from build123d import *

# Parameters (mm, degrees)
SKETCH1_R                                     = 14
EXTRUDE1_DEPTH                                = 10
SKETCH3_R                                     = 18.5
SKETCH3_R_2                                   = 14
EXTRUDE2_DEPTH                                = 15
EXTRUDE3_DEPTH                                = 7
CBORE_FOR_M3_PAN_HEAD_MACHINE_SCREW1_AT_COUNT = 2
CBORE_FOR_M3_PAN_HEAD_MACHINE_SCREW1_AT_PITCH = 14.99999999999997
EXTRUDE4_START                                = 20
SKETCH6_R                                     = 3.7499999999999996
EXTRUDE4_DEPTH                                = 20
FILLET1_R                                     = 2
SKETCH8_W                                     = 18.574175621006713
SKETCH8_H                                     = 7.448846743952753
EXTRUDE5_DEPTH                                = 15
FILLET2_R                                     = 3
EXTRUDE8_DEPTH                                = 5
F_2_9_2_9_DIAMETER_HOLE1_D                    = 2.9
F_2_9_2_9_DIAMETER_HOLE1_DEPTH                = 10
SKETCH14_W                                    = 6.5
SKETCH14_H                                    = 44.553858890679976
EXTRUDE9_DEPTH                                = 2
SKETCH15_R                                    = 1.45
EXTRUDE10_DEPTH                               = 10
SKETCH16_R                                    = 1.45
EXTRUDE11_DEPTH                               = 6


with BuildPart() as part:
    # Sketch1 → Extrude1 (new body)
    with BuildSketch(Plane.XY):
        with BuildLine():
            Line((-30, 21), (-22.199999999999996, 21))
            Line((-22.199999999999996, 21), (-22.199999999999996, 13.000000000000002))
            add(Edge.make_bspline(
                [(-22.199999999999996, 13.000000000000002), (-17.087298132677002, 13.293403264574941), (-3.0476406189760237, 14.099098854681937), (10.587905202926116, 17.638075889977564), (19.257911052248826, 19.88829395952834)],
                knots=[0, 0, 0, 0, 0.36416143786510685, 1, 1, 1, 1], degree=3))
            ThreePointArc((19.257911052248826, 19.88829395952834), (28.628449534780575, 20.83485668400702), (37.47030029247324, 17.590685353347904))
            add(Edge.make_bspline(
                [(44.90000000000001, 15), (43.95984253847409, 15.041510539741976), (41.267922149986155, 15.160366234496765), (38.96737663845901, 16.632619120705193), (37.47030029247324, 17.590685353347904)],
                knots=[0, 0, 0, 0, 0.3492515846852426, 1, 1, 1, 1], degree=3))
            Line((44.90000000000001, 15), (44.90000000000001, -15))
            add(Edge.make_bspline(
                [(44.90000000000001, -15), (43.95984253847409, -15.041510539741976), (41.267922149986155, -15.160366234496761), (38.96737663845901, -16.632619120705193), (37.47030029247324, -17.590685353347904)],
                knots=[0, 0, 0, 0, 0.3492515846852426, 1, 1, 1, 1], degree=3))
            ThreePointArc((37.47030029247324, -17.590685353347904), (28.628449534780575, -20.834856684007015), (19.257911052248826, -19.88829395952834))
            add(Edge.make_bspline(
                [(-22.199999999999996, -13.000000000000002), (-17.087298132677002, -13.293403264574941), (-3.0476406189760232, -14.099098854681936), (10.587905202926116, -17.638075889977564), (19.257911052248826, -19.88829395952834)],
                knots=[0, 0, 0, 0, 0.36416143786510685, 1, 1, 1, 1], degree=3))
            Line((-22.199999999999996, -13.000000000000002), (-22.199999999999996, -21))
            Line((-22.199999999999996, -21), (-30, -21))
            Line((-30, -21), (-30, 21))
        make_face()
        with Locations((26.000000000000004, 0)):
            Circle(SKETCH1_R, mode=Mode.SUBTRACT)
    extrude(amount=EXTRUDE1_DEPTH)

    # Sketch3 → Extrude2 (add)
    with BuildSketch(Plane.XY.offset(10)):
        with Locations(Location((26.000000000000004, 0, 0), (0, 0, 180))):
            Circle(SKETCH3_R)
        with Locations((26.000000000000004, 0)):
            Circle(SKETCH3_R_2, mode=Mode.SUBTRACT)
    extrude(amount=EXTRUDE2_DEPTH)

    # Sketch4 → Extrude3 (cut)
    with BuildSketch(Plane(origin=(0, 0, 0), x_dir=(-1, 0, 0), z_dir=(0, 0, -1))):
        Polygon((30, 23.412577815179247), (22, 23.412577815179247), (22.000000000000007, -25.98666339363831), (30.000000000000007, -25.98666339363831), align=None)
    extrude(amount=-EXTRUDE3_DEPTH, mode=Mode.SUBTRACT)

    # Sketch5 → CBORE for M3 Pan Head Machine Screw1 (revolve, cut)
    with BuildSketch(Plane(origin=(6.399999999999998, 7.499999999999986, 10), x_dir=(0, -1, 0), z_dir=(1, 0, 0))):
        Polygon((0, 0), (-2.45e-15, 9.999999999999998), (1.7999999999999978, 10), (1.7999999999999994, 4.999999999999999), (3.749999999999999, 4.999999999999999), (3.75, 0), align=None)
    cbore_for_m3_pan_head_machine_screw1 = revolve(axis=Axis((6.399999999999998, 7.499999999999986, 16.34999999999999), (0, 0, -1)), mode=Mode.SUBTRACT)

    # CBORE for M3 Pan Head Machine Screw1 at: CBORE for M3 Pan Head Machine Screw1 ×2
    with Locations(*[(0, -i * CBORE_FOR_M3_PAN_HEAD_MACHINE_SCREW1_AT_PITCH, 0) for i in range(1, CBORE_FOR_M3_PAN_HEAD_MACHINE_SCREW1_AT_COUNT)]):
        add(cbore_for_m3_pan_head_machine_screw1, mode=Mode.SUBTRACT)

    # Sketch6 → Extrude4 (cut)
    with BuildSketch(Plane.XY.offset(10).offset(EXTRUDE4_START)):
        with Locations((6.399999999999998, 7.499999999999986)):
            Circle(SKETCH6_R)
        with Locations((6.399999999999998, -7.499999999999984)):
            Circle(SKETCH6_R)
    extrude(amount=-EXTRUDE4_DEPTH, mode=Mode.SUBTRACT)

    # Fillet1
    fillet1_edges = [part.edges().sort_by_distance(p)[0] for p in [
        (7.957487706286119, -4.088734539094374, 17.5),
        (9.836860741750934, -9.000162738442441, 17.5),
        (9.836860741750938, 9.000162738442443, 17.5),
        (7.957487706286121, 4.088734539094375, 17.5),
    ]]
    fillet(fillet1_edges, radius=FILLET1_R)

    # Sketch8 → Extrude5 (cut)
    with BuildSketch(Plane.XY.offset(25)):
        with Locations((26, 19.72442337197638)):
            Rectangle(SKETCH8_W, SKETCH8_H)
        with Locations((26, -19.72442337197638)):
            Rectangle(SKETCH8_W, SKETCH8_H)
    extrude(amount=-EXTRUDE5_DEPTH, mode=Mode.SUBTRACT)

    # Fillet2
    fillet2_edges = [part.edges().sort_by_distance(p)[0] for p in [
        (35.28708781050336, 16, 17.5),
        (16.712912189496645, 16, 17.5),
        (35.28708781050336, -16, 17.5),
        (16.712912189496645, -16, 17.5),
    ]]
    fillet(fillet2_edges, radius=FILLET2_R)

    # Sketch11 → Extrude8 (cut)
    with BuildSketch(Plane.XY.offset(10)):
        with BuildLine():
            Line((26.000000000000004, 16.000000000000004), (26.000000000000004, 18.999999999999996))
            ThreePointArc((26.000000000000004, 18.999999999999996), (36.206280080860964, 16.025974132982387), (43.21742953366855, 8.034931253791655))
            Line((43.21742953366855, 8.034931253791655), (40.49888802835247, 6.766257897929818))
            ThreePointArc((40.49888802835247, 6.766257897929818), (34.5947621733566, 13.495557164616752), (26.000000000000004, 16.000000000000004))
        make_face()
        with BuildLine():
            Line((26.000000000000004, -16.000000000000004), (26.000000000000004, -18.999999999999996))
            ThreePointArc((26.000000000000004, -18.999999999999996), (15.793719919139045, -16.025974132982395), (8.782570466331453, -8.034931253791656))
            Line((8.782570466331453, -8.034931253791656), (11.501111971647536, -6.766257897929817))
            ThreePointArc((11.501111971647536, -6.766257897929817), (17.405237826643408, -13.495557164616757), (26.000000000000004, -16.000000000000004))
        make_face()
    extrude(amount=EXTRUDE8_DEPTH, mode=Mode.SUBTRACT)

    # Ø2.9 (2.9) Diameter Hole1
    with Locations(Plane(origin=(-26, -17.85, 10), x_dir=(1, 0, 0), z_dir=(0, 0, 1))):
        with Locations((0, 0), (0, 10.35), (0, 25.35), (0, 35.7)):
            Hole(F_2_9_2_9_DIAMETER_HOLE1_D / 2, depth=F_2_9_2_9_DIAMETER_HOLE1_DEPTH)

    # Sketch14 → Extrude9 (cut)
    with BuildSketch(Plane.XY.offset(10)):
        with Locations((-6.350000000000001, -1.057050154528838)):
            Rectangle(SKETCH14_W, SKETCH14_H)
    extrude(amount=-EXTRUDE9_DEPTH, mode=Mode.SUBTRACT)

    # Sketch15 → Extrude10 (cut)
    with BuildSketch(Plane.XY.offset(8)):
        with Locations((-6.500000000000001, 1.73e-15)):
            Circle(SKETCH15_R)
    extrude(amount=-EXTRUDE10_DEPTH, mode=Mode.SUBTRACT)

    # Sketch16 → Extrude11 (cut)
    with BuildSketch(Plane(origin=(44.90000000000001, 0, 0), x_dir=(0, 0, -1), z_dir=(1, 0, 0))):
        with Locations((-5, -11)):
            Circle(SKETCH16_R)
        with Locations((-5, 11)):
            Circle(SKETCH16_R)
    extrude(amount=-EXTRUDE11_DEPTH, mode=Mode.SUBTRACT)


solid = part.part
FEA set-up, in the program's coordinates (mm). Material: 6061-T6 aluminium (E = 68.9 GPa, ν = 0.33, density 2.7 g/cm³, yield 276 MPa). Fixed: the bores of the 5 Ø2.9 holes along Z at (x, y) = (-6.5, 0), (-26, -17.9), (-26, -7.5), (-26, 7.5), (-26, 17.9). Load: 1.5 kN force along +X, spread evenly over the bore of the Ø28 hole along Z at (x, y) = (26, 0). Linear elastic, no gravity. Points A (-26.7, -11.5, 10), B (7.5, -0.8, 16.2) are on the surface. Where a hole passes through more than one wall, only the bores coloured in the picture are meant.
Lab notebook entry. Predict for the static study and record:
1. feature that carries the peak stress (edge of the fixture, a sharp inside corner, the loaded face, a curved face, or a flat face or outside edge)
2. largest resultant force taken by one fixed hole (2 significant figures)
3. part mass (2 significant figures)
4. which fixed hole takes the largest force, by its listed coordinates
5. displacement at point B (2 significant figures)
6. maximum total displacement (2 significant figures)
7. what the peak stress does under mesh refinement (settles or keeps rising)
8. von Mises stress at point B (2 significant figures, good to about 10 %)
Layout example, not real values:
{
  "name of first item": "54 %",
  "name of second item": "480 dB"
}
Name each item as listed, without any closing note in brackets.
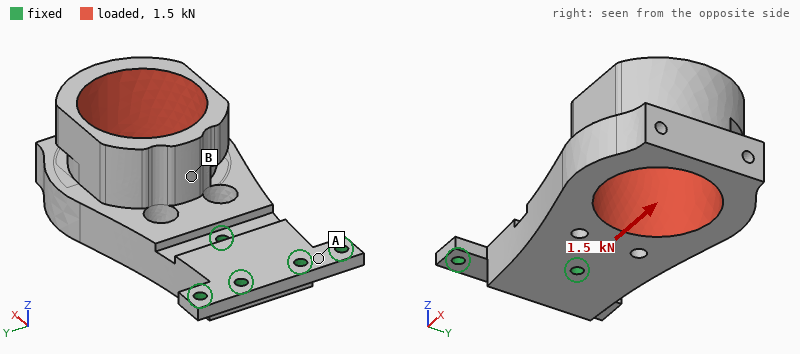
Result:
{
  "feature that carries the peak stress": "edge of the fixture",
  "largest resultant force taken by one fixed hole": "1.1 kN",
  "part mass": "59 g",
  "which fixed hole takes the largest force, by its listed coordinates": "(-6.5, 0)",
  "displacement at point B": "0.035 mm",
  "maximum total displacement": "0.15 mm",
  "what the peak stress does under mesh refinement": "keeps rising",
  "von Mises stress at point B": "12 MPa"
}
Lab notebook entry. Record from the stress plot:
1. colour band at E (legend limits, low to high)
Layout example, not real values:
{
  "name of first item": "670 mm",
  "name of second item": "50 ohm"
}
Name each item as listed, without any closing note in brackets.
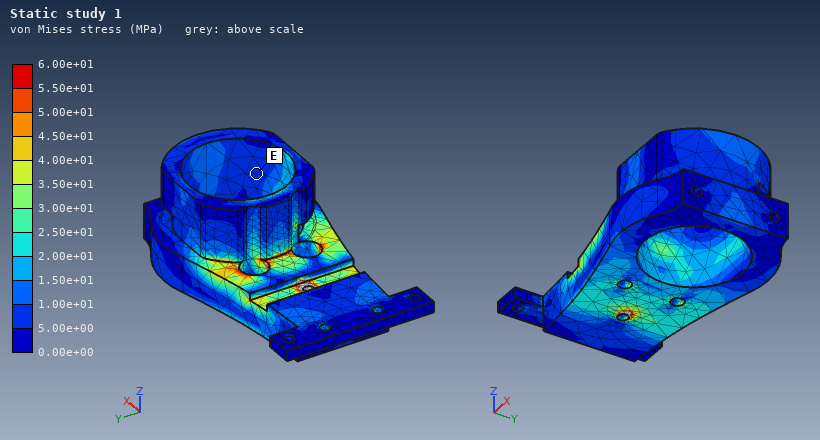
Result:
{
  "colour band at E": "5.00e+00 to 1.00e+01 MPa"
}
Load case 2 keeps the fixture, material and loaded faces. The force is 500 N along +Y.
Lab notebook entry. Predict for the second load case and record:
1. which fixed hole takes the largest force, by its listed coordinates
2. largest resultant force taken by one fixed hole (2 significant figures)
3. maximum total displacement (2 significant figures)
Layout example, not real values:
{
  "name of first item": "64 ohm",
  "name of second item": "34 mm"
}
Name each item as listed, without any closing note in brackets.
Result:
{
  "which fixed hole takes the largest force, by its listed coordinates": "(-6.5, 0)",
  "largest resultant force taken by one fixed hole": "1.0 kN",
  "maximum total displacement": "60 µm"
}
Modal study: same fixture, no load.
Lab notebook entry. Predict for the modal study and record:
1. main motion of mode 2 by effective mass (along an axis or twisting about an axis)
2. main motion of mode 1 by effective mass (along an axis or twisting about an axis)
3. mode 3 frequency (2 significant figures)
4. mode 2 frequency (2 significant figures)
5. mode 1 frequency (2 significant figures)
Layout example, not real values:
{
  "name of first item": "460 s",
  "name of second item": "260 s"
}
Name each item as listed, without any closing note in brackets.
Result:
{
  "main motion of mode 2 by effective mass": "along Y",
  "main motion of mode 1 by effective mass": "along Z",
  "mode 3 frequency": "4300 Hz",
  "mode 2 frequency": "3000 Hz",
  "mode 1 frequency": "1800 Hz"
}
